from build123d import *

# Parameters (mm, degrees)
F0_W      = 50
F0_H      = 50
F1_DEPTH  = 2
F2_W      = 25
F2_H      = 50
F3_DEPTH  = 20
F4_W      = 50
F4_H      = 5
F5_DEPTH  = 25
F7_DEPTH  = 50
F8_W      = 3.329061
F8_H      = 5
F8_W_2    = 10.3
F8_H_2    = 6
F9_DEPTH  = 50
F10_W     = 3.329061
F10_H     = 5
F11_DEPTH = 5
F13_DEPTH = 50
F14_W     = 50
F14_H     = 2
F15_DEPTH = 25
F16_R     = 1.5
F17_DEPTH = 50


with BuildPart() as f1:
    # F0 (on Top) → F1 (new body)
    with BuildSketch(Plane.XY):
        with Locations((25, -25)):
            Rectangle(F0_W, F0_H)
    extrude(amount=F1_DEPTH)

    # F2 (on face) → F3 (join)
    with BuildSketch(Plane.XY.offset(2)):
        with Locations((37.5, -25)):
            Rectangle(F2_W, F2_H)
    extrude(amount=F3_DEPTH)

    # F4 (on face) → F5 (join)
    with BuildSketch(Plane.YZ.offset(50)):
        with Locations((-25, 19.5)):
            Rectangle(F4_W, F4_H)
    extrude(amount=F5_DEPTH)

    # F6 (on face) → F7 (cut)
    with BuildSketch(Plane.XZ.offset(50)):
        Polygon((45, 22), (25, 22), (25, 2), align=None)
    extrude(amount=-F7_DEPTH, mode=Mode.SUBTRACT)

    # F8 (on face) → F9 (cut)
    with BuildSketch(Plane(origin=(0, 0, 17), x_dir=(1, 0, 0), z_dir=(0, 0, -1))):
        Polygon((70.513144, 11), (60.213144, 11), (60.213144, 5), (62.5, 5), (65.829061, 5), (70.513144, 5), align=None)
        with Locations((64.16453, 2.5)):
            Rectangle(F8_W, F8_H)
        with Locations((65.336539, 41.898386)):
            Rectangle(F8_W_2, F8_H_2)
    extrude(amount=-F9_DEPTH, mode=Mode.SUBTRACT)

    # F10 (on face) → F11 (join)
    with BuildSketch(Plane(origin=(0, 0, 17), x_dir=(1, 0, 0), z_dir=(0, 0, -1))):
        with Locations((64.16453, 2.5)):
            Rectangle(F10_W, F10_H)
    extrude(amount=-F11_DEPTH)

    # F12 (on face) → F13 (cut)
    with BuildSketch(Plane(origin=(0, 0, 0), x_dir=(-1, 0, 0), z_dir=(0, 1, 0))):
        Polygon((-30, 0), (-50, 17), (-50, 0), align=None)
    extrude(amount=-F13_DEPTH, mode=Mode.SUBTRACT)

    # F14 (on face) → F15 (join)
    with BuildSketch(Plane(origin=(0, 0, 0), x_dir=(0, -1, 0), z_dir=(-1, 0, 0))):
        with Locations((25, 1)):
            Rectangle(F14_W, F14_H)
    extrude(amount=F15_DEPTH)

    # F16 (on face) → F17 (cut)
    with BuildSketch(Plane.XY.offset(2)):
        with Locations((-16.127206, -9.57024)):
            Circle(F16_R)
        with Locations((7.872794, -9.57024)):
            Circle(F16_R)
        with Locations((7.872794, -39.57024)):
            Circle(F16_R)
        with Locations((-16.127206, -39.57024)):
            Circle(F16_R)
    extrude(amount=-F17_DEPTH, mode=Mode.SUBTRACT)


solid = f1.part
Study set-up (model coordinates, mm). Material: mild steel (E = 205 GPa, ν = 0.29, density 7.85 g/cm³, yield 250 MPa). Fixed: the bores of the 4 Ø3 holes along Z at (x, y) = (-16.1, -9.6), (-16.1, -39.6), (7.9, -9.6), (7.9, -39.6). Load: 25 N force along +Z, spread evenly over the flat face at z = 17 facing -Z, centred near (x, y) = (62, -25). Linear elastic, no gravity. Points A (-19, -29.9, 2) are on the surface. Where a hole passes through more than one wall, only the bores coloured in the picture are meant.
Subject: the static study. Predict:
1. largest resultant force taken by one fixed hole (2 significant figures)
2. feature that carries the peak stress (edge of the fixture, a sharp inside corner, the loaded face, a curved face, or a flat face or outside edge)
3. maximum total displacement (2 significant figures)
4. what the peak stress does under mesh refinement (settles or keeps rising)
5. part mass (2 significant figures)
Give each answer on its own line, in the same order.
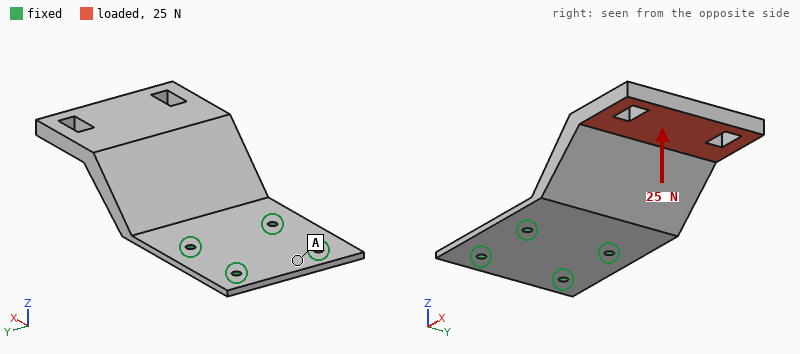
22 N
edge of the fixture
0.19 mm
keeps rising
150 g
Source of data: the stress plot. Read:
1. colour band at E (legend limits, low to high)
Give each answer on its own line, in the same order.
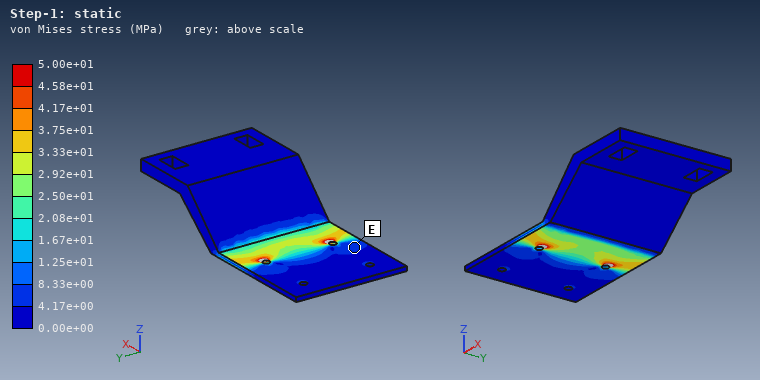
4.17e+00 to 8.33e+00 MPa
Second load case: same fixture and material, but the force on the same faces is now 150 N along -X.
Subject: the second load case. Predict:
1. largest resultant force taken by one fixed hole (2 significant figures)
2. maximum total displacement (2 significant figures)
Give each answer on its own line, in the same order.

64 N
0.40 mm
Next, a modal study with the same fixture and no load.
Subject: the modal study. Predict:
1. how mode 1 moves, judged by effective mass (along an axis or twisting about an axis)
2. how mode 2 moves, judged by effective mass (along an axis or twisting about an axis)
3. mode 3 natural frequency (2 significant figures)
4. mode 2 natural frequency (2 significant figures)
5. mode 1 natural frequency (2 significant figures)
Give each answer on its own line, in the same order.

along Z
along Y
2600 Hz
1100 Hz
240 Hz
